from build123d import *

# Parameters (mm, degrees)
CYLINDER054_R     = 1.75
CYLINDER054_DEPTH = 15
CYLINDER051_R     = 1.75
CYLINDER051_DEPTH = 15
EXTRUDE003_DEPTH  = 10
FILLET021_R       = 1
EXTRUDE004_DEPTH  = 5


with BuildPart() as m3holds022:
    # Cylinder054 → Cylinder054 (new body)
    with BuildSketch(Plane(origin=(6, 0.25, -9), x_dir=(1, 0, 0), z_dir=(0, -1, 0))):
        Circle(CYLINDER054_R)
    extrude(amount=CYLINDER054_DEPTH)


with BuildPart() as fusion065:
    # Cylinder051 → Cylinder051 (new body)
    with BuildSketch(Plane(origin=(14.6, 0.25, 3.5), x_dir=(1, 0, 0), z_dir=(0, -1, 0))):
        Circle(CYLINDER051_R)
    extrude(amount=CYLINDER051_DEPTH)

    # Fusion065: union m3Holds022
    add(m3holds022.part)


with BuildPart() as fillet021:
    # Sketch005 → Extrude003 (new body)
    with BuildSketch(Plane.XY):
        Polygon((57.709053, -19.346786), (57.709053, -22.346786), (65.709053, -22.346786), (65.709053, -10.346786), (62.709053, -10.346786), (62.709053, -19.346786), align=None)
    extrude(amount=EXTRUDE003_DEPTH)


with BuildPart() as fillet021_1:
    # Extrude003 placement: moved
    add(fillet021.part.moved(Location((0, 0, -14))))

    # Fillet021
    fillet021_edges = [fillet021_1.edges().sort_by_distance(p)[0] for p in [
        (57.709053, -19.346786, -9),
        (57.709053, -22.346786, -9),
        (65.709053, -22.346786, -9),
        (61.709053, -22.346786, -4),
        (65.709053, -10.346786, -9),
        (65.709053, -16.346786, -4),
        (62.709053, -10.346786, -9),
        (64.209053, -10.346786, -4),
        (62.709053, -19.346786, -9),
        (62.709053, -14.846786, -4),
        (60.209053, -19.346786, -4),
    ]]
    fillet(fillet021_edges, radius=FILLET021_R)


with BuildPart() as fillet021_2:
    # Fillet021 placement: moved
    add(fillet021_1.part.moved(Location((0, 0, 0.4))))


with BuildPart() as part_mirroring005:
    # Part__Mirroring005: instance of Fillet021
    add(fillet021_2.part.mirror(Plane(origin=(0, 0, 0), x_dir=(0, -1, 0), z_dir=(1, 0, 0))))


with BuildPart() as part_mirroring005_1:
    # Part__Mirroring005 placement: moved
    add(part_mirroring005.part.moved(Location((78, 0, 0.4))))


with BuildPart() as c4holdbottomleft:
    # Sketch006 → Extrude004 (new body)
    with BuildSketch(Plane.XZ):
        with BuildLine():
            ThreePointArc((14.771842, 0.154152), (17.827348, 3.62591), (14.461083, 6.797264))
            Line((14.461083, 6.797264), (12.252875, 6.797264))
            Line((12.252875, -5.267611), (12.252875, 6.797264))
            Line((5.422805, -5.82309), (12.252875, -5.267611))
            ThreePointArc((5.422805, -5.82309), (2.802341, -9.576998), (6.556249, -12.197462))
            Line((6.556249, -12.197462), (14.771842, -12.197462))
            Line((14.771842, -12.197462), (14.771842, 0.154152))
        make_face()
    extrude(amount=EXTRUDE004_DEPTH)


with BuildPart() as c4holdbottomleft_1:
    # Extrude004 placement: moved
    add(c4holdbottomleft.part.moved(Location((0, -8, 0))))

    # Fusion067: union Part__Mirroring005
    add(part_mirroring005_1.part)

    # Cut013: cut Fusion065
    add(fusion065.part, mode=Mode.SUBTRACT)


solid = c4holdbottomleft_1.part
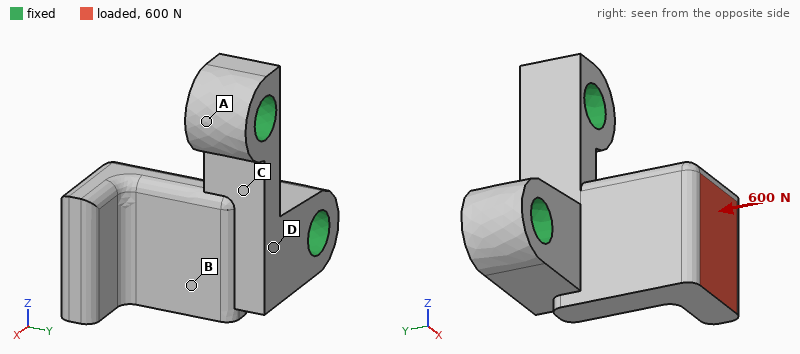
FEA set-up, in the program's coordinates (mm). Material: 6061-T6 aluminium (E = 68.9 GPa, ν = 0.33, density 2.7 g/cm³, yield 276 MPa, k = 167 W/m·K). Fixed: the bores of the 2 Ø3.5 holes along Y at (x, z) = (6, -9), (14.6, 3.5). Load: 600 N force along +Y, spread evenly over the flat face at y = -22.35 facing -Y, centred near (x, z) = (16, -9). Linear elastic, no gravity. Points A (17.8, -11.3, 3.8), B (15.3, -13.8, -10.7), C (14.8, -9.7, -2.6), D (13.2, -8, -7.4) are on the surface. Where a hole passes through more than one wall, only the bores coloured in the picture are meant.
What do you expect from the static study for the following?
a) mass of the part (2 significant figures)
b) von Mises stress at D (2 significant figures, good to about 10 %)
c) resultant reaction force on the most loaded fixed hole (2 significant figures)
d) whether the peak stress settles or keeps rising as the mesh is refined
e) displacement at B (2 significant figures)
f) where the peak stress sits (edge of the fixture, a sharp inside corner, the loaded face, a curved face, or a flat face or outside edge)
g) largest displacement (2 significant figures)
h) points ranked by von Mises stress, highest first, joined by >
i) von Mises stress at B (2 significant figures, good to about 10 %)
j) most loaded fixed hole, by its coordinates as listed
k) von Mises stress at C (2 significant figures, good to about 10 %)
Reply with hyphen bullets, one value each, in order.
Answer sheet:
- 2.6 g
- 34 MPa
- 410 N
- keeps rising
- 0.036 mm
- edge of the fixture
- 0.15 mm
- B > C > D > A
- 120 MPa
- (6, -9)
- 86 MPa
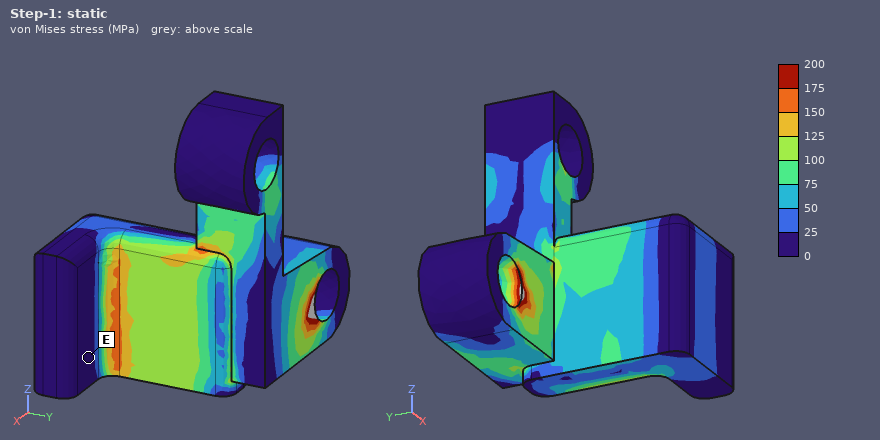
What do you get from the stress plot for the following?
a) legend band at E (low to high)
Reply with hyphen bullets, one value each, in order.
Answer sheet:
- 0 to 25 MPa
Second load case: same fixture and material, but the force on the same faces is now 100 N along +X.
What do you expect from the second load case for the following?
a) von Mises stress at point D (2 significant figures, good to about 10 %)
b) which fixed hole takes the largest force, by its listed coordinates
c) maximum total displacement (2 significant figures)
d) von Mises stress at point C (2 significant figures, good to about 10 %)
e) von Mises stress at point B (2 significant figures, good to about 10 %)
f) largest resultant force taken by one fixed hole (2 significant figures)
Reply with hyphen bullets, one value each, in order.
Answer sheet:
- 12 MPa
- (6, -9)
- 55 µm
- 25 MPa
- 54 MPa
- 120 N
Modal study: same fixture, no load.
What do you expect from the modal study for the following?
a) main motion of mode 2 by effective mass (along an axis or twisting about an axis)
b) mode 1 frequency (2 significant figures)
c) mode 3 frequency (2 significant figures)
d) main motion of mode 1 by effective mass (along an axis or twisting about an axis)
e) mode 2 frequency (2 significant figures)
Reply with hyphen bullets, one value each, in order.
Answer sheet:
- along Z
- 9500 Hz
- 26 kHz
- along X
- 17 kHz
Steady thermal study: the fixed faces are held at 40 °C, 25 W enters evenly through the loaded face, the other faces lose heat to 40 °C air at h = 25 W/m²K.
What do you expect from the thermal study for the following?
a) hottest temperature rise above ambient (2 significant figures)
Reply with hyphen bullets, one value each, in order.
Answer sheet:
- 74 K
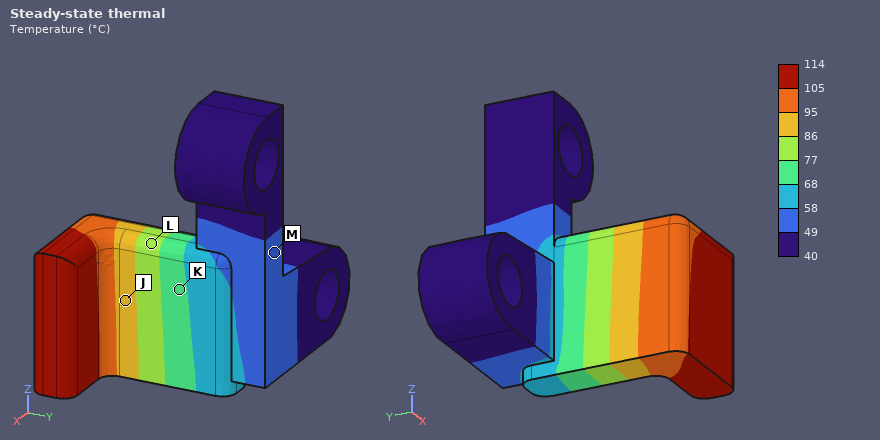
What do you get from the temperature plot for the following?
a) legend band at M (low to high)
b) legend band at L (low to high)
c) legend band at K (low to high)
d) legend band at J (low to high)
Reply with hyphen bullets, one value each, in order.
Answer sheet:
- 49 to 58 °C
- 77 to 86 °C
- 68 to 77 °C
- 86 to 95 °C
